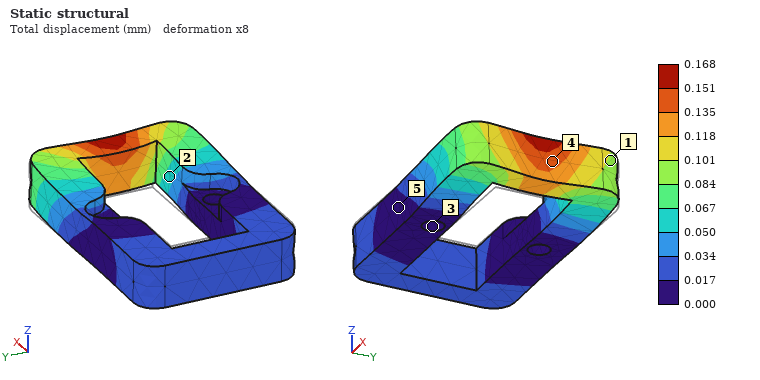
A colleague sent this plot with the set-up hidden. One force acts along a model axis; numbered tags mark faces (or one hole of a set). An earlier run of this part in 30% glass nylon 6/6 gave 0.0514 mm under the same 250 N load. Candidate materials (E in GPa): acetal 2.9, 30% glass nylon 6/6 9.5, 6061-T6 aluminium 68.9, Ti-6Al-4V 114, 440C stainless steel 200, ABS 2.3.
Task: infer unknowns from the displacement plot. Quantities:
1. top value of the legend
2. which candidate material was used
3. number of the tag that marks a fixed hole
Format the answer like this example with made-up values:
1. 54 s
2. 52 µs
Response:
1. 0.168 mm
2. acetal
3. 3
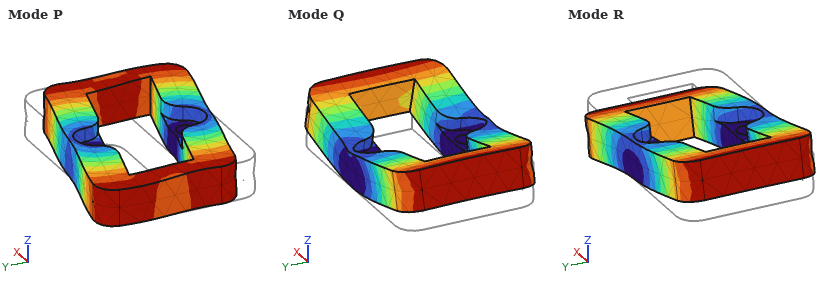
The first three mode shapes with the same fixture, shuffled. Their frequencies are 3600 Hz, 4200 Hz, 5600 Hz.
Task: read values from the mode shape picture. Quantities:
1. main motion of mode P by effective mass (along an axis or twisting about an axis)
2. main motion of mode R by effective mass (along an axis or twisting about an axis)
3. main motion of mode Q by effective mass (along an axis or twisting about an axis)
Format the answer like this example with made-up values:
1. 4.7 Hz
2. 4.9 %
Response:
1. twisting about Z
2. twisting about Y
3. along Z
